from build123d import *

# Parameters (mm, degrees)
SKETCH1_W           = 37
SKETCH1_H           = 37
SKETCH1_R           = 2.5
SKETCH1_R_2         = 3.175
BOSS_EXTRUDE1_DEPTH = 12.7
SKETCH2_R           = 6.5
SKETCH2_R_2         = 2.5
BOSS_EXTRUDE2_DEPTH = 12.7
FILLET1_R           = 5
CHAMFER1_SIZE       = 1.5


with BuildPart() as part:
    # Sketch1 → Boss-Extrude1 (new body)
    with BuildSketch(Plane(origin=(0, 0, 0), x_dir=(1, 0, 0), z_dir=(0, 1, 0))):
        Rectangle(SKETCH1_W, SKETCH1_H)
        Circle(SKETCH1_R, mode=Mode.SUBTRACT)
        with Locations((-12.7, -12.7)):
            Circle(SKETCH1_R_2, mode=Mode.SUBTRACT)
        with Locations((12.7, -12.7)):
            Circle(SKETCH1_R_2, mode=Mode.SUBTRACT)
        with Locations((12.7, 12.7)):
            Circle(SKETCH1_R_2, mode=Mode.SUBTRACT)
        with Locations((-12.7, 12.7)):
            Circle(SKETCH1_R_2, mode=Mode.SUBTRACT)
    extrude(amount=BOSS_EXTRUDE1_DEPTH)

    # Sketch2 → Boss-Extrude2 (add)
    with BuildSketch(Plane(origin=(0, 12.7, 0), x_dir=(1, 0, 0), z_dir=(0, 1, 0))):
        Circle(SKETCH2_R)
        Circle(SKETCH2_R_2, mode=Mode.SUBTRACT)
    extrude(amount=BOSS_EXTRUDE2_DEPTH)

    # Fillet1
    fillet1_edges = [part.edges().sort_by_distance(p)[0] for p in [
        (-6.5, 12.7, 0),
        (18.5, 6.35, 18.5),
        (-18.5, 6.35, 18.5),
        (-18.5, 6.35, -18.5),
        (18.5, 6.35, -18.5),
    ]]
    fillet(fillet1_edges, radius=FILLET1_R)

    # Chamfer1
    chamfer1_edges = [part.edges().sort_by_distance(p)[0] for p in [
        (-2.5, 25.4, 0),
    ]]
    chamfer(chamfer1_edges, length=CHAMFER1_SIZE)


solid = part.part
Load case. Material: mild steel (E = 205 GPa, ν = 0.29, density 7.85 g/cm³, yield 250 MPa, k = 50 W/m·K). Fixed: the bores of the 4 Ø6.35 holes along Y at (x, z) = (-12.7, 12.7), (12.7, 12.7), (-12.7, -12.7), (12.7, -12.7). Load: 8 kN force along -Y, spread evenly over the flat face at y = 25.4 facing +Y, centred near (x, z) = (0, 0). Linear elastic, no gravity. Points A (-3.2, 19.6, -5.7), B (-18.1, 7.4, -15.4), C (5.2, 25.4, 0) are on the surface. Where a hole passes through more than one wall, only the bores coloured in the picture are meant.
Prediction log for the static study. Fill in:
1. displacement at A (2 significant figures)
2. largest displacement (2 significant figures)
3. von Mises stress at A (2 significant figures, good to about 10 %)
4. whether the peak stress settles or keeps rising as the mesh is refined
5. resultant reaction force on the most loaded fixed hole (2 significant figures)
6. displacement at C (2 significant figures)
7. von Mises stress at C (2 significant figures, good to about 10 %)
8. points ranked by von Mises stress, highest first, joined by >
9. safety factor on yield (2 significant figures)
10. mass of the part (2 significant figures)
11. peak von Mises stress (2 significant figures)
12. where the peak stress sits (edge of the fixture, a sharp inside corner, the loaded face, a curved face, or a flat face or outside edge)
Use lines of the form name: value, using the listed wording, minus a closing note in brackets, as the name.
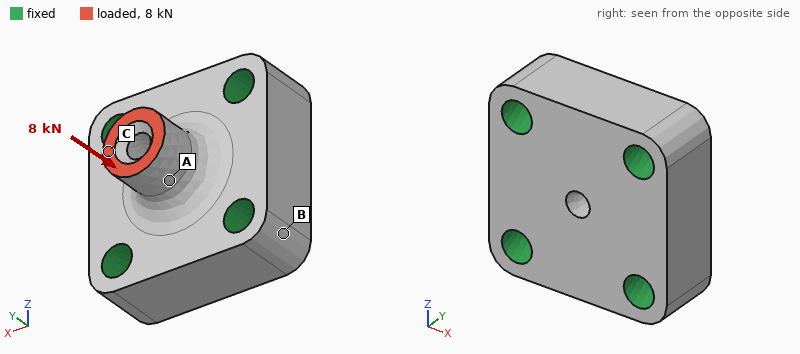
displacement at A: 4.4 µm
largest displacement: 7.3 µm
von Mises stress at A: 81 MPa
whether the peak stress settles or keeps rising as the mesh is refined: settles
resultant reaction force on the most loaded fixed hole: 2.1 kN
displacement at C: 6.8 µm
von Mises stress at C: 100 MPa
points ranked by von Mises stress, highest first, joined by >: C > A > B
safety factor on yield: 2.1
mass of the part: 130 g
peak von Mises stress: 120 MPa
where the peak stress sits: the loaded face
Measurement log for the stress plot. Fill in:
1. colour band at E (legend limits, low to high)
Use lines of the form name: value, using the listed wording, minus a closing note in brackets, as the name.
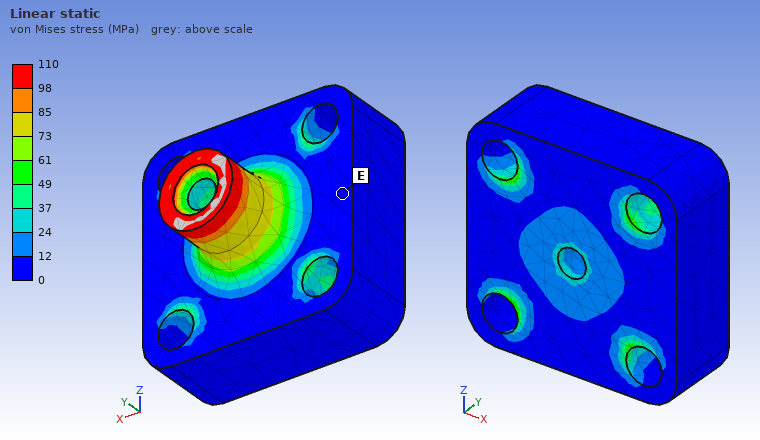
colour band at E: 0 to 12 MPa
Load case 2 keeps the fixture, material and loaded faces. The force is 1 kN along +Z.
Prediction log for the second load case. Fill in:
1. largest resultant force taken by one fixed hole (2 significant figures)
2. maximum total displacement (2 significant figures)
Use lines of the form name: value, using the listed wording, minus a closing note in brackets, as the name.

largest resultant force taken by one fixed hole: 480 N
maximum total displacement: 5.5 µm
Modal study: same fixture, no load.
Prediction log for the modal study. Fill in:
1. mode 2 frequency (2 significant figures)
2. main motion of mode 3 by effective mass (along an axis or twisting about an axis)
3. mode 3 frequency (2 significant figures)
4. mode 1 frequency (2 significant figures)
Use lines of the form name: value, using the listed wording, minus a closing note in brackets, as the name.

mode 2 frequency: 37 kHz
main motion of mode 3 by effective mass: along Y
mode 3 frequency: 44 kHz
mode 1 frequency: 37 kHz
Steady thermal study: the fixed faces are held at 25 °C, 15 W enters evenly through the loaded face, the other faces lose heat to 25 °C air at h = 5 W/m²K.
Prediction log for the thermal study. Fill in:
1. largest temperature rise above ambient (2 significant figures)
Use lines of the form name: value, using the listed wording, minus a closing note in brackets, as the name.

largest temperature rise above ambient: 40 K
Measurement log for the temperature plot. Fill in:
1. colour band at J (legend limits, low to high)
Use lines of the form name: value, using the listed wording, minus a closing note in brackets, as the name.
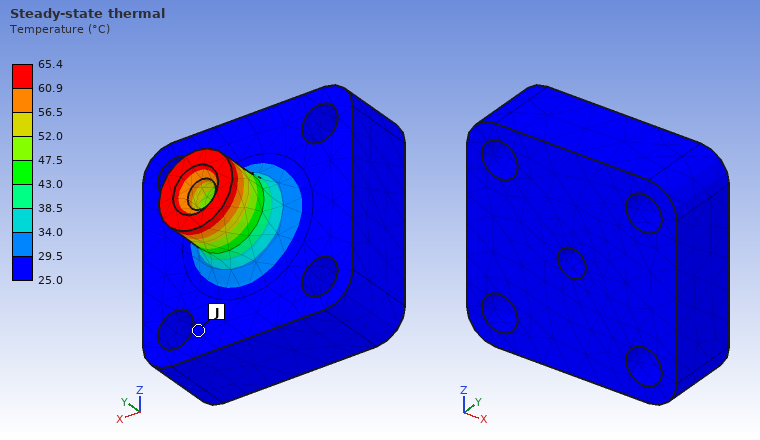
colour band at J: 25.0 to 29.5 °C
